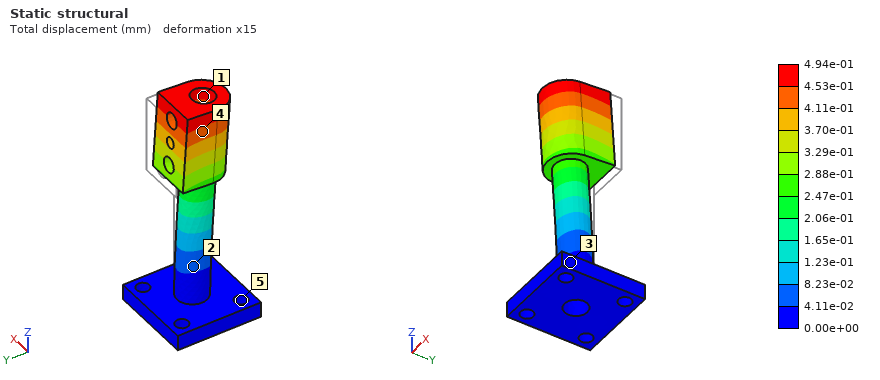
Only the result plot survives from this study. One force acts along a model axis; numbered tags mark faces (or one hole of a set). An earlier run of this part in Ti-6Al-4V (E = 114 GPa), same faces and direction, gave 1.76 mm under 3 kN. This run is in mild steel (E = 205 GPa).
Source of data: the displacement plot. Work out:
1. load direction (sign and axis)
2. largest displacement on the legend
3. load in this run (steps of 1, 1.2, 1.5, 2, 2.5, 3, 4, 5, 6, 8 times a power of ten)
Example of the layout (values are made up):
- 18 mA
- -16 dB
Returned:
- -Y
- 4.94e-01 mm
- 1.5 kN
